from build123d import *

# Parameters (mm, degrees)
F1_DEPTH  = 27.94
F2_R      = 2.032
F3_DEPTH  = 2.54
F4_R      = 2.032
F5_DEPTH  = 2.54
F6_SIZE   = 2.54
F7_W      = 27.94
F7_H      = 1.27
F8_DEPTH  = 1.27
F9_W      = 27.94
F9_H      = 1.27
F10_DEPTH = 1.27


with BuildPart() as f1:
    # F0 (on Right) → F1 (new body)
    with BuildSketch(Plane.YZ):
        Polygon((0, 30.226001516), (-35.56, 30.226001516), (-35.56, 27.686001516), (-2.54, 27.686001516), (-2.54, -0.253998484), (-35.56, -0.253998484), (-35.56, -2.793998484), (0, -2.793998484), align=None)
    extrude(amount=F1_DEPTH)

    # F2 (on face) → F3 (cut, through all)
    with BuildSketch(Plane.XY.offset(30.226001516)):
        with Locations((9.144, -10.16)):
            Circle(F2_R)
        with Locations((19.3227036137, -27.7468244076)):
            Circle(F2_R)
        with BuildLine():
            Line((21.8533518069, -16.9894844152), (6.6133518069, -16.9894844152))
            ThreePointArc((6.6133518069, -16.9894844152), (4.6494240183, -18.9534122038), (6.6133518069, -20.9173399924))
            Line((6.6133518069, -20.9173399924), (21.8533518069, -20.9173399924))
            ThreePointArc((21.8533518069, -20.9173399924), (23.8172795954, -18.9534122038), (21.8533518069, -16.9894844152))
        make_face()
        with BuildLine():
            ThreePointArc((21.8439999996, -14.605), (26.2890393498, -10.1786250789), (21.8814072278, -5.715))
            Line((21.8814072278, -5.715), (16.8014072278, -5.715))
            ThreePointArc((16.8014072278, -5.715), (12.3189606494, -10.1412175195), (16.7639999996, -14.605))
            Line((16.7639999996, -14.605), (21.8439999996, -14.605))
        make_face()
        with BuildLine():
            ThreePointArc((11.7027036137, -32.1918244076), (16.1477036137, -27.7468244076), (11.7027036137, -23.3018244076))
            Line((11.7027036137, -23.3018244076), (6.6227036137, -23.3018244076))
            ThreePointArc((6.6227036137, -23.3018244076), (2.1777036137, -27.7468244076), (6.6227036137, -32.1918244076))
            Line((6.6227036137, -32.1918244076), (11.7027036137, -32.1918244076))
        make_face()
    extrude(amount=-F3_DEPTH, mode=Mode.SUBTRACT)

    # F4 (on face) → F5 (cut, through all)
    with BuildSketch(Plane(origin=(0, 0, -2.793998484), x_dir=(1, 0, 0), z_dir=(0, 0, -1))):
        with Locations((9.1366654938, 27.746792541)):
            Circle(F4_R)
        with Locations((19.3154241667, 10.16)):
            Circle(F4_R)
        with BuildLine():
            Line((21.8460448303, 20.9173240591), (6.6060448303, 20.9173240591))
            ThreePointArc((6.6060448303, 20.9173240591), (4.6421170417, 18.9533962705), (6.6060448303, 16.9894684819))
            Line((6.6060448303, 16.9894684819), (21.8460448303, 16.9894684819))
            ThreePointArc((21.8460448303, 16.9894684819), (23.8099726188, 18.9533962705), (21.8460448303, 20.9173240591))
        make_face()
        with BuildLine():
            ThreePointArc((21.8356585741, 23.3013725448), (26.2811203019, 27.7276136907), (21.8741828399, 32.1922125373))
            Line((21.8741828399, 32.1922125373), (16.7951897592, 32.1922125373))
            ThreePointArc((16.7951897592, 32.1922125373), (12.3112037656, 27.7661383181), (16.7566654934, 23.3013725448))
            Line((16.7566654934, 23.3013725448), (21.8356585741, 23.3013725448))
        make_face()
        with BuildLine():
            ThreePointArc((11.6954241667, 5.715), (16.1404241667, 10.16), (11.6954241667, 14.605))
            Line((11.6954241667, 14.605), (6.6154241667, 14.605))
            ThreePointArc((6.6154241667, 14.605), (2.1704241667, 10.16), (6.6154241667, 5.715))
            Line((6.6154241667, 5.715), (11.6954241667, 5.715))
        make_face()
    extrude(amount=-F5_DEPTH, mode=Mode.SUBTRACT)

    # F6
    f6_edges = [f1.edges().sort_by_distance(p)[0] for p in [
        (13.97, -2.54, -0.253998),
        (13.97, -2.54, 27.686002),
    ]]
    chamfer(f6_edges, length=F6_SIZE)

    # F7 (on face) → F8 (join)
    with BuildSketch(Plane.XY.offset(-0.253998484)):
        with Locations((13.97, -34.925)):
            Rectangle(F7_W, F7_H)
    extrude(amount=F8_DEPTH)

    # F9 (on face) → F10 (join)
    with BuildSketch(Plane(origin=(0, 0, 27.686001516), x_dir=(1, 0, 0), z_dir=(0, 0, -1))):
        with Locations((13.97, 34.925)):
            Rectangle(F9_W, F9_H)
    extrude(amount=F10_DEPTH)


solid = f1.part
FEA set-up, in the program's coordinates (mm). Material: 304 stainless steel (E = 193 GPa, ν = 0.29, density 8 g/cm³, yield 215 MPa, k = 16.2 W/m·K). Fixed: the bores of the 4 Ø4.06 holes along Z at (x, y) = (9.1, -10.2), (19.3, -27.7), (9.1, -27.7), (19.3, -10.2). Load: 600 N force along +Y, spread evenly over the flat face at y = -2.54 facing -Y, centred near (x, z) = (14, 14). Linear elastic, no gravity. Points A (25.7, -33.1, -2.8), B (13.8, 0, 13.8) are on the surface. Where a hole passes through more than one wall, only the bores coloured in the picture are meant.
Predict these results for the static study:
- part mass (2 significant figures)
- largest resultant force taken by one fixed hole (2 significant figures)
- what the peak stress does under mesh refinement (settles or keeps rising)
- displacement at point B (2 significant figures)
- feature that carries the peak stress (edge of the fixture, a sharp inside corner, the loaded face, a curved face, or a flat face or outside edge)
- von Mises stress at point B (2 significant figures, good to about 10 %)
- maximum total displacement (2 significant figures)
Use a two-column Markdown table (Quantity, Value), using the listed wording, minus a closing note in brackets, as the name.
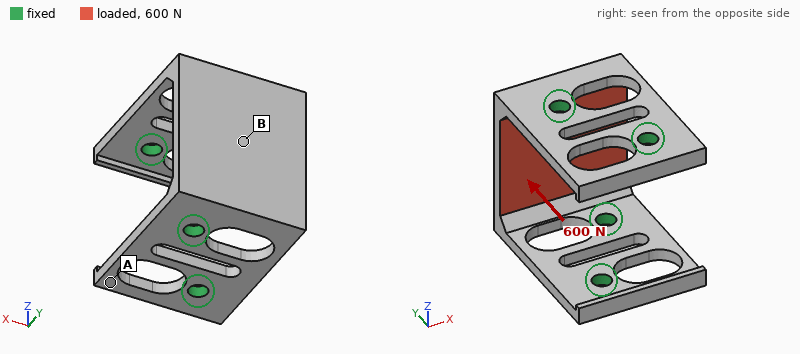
| Quantity | Value |
|---|---|
| part mass | 46 g |
| largest resultant force taken by one fixed hole | 380 N |
| what the peak stress does under mesh refinement | keeps rising |
| displacement at point B | 9.0 µm |
| feature that carries the peak stress | edge of the fixture |
| von Mises stress at point B | 37 MPa |
| maximum total displacement | 11 µm |
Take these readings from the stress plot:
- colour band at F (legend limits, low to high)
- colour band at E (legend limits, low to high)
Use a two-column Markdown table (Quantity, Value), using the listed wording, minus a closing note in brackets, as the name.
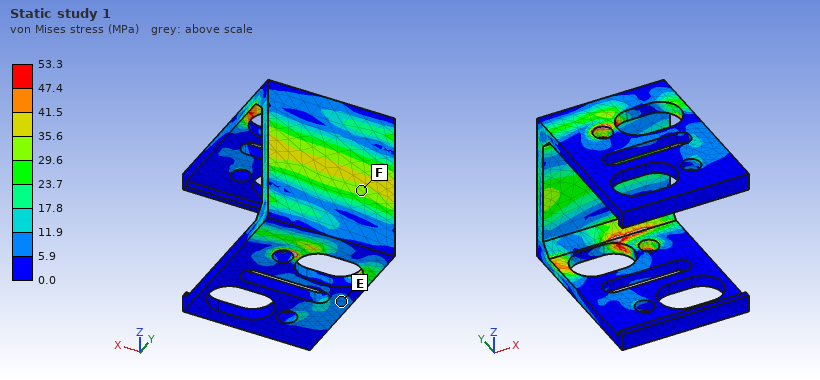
| Quantity | Value |
|---|---|
| colour band at F | 29.6 to 35.6 MPa |
| colour band at E | 5.9 to 11.9 MPa |
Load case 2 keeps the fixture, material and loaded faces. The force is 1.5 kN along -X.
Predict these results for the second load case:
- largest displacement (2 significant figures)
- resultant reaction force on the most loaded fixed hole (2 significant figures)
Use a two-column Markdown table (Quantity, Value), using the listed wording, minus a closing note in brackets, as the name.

| Quantity | Value |
|---|---|
| largest displacement | 6.6 µm |
| resultant reaction force on the most loaded fixed hole | 850 N |
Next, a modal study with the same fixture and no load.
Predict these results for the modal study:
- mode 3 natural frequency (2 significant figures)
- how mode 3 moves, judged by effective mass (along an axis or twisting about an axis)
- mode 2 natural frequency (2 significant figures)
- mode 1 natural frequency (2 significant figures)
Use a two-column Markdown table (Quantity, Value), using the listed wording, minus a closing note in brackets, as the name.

| Quantity | Value |
|---|---|
| mode 3 natural frequency | 10 kHz |
| how mode 3 moves, judged by effective mass | along Z |
| mode 2 natural frequency | 7400 Hz |
| mode 1 natural frequency | 7100 Hz |
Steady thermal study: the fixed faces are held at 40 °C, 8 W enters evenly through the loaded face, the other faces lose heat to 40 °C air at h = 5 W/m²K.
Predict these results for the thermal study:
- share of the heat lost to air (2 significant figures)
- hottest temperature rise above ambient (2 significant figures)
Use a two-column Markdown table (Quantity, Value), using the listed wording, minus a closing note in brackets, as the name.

| Quantity | Value |
|---|---|
| share of the heat lost to air | 7.5 % |
| hottest temperature rise above ambient | 76 K |
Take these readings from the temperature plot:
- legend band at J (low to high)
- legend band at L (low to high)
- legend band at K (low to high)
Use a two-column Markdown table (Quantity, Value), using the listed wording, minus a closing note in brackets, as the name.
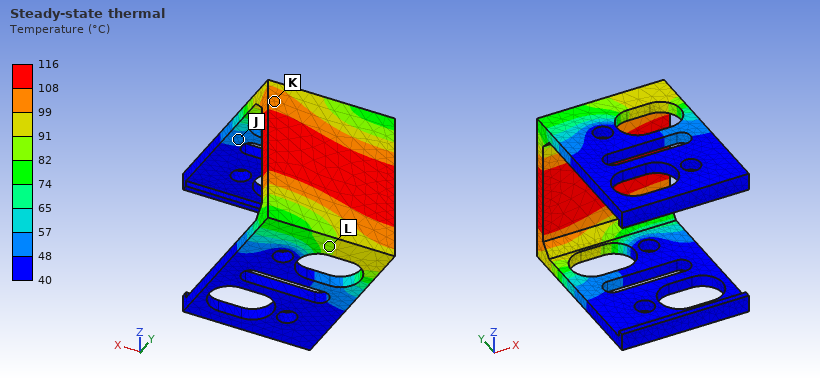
| Quantity | Value |
|---|---|
| legend band at J | 48 to 57 °C |
| legend band at L | 82 to 91 °C |
| legend band at K | 99 to 108 °C |
